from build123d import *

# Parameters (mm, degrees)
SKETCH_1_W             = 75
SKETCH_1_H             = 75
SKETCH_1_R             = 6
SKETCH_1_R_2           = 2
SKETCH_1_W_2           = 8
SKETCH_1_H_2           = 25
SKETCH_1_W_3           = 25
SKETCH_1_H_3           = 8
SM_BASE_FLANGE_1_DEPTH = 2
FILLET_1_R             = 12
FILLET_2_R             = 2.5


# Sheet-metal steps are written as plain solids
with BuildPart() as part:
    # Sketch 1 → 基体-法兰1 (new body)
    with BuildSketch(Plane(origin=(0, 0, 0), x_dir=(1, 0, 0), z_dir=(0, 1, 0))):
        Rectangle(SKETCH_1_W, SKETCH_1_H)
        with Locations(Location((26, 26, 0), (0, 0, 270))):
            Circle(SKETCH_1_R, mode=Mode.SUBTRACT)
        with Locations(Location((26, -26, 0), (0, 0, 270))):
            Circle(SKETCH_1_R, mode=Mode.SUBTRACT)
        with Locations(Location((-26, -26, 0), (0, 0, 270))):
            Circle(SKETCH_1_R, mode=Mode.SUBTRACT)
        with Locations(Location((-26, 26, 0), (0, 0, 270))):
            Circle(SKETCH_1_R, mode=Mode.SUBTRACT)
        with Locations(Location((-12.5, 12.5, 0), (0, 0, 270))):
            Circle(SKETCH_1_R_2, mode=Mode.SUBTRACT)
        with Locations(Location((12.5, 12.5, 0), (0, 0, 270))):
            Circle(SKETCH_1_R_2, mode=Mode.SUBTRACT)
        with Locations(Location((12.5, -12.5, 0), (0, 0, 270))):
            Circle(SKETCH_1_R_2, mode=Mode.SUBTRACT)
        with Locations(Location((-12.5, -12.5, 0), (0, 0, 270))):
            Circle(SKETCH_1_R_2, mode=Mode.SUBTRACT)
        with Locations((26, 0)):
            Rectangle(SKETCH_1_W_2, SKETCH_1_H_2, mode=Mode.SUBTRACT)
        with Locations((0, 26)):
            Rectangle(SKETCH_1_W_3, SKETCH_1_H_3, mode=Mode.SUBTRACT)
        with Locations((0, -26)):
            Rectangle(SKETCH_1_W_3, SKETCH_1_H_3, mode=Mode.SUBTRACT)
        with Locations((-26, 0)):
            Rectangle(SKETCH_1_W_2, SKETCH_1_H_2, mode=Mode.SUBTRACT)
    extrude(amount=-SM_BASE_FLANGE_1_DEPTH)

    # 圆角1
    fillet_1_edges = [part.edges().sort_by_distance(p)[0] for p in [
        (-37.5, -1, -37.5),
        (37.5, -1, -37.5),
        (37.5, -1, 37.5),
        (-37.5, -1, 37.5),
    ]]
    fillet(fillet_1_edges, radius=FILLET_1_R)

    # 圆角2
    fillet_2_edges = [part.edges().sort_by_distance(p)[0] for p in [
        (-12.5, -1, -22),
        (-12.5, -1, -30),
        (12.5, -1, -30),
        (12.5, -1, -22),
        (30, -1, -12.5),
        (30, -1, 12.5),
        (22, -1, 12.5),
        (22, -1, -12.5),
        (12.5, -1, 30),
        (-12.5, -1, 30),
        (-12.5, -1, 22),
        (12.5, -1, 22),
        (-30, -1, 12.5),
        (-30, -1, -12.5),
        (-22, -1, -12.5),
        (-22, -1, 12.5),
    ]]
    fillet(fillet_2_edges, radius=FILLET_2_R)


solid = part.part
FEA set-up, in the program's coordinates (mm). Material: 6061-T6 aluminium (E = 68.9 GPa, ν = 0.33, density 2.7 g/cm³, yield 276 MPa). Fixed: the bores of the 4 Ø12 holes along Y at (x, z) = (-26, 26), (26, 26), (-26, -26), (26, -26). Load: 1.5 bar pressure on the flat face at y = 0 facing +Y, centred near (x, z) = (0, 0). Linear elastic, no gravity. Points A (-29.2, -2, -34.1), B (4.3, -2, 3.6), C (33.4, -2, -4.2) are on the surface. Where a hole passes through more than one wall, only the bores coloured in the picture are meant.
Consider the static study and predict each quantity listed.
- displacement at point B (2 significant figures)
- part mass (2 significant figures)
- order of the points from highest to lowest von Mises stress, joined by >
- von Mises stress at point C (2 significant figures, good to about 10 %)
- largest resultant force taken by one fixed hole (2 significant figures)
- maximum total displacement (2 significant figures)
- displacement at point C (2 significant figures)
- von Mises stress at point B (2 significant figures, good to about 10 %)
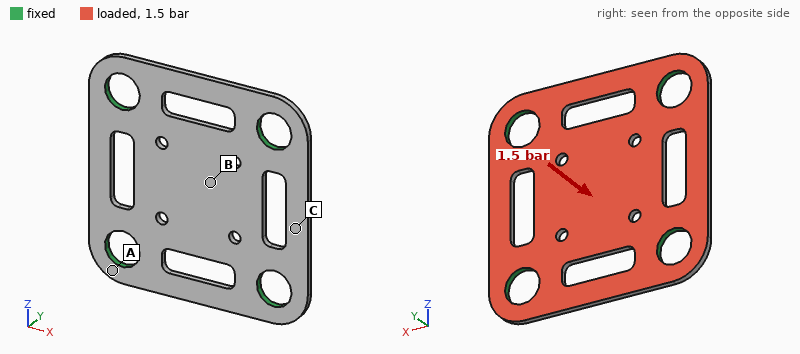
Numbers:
69 µm
23 g
B > C > A
12 MPa
160 N
73 µm
22 µm
21 MPa
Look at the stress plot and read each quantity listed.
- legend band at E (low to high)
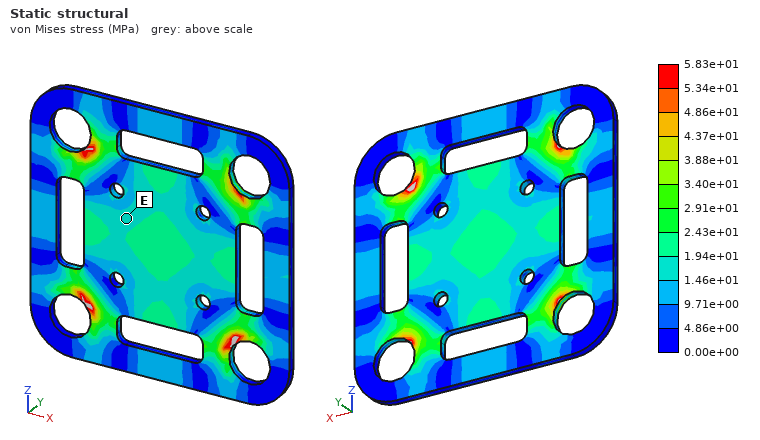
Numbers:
1.46e+01 to 1.94e+01 MPa
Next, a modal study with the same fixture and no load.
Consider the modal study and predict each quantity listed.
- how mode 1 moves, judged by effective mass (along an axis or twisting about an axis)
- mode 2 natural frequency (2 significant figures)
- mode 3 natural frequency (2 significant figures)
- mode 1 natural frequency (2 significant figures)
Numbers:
along Y
6300 Hz
6300 Hz
3700 Hz
